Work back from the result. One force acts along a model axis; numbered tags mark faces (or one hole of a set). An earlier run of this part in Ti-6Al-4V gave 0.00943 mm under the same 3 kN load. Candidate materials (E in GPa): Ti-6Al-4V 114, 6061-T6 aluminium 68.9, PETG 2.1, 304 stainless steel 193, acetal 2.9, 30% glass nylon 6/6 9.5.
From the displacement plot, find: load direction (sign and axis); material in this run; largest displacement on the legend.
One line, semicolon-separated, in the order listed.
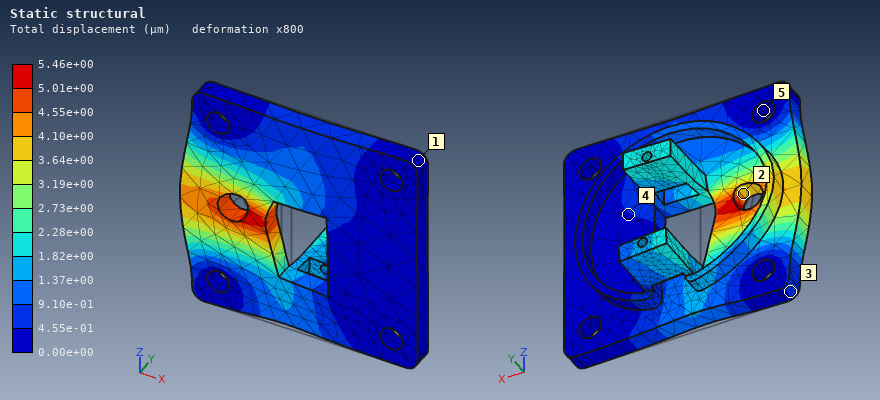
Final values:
-X; 304 stainless steel; 5.46e+00 µm
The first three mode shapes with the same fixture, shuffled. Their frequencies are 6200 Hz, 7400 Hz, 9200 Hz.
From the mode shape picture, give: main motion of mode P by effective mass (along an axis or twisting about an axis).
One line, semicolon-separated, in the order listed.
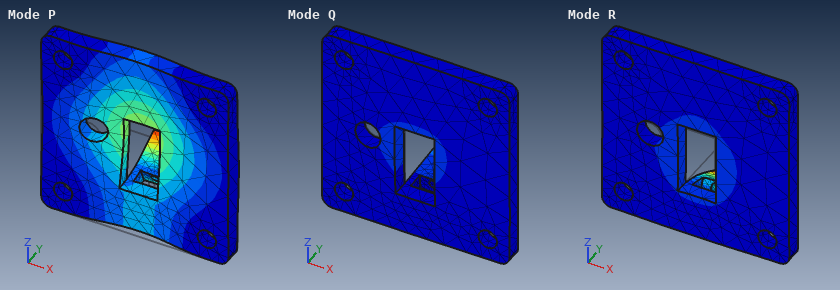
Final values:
along Y
